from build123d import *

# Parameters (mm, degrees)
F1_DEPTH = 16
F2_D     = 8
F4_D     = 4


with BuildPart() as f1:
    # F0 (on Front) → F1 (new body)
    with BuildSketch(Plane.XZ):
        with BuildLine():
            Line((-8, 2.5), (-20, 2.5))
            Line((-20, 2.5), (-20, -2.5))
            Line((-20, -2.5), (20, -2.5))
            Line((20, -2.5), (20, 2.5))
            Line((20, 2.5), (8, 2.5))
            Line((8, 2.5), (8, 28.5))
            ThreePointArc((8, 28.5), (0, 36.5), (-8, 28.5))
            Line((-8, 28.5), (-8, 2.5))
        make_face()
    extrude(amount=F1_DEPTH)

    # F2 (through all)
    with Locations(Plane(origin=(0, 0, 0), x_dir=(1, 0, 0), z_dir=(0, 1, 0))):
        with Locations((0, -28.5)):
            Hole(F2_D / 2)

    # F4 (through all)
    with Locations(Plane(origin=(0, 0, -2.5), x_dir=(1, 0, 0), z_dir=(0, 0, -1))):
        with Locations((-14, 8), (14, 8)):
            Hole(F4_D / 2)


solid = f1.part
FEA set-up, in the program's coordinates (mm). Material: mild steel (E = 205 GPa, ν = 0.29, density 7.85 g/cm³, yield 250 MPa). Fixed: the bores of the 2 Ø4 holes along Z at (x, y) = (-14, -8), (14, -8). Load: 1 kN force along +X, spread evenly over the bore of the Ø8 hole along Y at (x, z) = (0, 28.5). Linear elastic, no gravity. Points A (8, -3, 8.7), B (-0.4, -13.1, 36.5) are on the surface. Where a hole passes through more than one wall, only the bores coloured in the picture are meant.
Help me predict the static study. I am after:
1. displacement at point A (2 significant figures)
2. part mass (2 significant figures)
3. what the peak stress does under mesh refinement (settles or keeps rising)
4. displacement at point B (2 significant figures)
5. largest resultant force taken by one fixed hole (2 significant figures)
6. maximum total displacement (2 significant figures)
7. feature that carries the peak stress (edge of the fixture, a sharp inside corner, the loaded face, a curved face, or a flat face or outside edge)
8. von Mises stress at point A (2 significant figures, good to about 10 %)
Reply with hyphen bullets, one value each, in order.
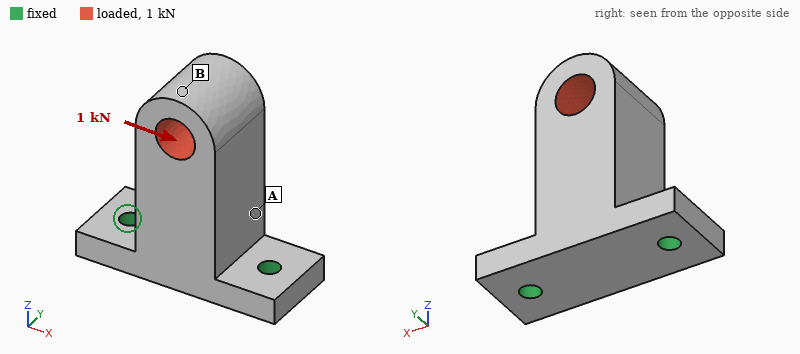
- 5.4 µm
- 83 g
- keeps rising
- 23 µm
- 1.4 kN
- 23 µm
- edge of the fixture
- 29 MPa
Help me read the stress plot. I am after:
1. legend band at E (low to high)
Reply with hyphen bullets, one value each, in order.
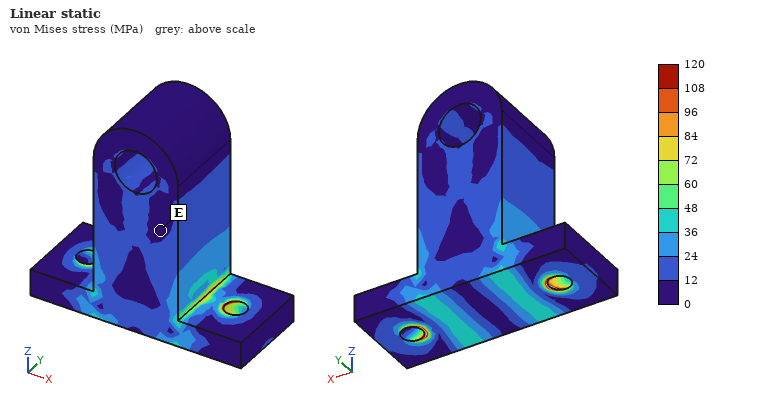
- 0 to 12 MPa
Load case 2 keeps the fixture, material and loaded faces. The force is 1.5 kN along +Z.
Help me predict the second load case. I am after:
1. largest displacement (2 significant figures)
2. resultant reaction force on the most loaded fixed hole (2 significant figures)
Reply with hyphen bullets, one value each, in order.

- 3.5 µm
- 790 N
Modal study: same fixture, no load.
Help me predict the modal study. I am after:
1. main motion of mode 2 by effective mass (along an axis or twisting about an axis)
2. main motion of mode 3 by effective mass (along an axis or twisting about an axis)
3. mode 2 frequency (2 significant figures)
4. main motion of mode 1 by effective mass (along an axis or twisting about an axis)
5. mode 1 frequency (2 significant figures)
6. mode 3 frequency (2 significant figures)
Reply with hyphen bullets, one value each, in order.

- along X
- along Z
- 7300 Hz
- along Y
- 3600 Hz
- 15 kHz
